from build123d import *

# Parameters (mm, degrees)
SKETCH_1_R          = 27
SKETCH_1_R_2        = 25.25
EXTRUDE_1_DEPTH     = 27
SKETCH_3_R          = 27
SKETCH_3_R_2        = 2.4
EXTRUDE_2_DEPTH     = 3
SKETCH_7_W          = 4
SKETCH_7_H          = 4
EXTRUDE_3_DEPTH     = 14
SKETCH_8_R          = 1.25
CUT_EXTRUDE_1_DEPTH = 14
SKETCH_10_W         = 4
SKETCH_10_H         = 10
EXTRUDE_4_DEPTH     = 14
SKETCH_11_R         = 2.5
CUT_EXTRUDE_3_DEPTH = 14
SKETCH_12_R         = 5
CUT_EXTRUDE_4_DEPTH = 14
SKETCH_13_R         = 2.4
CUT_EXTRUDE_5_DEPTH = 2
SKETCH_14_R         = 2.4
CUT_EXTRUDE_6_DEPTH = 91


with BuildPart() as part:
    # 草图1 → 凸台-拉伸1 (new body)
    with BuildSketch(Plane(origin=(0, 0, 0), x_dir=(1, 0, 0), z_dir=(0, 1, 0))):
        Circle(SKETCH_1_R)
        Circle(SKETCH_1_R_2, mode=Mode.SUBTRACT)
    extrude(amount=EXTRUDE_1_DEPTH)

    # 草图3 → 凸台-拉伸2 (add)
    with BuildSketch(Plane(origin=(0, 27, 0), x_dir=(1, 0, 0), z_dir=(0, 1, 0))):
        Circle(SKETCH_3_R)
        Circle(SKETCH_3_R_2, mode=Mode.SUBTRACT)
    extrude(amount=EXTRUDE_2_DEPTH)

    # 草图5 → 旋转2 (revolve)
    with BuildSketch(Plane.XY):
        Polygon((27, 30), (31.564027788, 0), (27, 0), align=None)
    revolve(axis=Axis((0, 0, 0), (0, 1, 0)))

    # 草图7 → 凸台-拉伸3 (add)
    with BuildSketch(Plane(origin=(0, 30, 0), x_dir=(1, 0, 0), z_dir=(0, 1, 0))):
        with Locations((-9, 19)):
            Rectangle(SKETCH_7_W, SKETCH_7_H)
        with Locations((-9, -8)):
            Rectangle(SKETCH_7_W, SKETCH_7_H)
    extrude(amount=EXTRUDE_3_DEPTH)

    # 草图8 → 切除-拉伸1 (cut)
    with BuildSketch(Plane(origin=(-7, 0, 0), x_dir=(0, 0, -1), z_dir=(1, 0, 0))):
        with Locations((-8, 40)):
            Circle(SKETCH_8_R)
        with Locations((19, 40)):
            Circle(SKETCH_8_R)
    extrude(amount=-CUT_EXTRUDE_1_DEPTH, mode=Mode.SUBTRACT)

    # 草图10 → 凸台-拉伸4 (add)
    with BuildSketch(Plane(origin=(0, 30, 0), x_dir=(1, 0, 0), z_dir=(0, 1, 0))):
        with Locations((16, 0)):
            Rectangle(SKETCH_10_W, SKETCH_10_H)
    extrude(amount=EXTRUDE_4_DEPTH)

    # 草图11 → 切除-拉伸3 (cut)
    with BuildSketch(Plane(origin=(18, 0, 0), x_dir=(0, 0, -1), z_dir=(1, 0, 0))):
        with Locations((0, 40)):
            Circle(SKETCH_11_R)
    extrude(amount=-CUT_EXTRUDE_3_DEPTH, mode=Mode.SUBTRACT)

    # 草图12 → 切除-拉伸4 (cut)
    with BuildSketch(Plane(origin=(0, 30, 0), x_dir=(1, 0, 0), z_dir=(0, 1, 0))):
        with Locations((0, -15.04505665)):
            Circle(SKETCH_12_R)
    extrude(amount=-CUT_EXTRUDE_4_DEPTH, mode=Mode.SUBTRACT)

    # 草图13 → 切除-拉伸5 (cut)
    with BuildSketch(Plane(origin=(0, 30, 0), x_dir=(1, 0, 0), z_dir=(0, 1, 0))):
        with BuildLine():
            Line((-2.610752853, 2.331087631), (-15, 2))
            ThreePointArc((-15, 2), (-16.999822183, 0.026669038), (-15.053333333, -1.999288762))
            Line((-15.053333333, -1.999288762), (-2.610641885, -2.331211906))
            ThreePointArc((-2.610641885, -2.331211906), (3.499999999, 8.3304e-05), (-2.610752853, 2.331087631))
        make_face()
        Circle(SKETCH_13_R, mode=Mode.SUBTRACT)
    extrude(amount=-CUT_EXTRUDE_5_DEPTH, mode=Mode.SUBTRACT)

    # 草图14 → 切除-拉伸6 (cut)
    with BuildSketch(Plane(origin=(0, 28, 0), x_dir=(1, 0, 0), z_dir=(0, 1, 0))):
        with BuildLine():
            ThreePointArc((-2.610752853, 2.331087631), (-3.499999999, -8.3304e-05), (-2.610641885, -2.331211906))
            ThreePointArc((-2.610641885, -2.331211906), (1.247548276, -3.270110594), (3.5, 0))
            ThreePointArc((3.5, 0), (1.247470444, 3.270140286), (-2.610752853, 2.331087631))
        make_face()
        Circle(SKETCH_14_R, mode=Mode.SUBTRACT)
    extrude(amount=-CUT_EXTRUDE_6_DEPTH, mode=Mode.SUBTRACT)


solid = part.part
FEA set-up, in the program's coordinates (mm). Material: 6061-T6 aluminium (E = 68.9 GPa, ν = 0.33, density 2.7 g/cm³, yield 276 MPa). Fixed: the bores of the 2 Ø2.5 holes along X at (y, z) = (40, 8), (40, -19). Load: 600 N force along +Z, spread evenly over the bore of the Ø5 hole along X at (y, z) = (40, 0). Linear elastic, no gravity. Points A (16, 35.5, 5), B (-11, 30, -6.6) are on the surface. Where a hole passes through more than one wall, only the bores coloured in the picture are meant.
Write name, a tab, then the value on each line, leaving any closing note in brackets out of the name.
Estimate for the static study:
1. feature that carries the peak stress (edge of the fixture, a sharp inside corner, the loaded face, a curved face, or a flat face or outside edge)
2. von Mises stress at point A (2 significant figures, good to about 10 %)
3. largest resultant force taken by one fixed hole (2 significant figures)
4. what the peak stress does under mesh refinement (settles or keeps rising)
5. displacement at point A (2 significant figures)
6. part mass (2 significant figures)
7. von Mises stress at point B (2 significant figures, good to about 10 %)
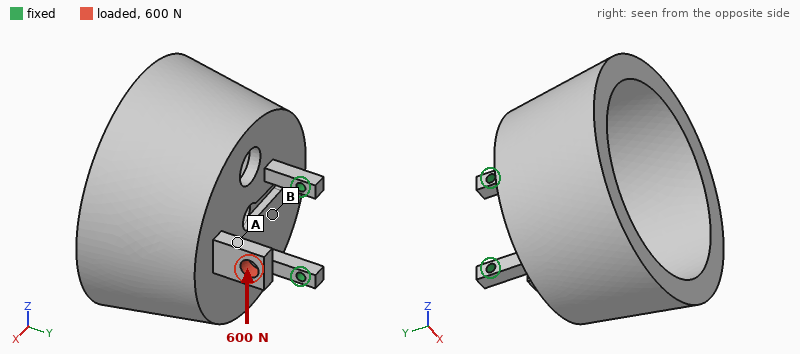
feature that carries the peak stress	edge of the fixture
von Mises stress at point A	58 MPa
largest resultant force taken by one fixed hole	620 N
what the peak stress does under mesh refinement	keeps rising
displacement at point A	0.18 mm
part mass	74 g
von Mises stress at point B	20 MPa
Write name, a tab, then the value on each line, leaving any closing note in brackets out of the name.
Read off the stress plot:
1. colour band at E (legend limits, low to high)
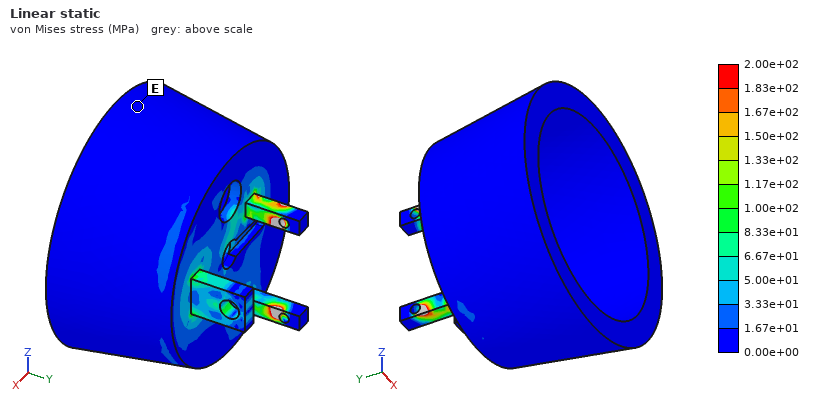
colour band at E	0.00e+00 to 1.67e+01 MPa
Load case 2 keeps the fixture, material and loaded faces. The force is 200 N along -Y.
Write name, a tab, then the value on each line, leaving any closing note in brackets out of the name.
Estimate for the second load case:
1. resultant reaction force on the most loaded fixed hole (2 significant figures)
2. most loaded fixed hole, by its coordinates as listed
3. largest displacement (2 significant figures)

resultant reaction force on the most loaded fixed hole	140 N
most loaded fixed hole, by its coordinates as listed	(40, 8)
largest displacement	1.0 mm
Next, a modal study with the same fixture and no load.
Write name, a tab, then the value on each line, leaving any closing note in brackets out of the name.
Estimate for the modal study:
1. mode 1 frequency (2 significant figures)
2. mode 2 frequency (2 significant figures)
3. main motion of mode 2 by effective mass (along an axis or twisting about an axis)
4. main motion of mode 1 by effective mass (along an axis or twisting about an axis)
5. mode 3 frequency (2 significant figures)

mode 1 frequency	330 Hz
mode 2 frequency	1100 Hz
main motion of mode 2 by effective mass	along Z
main motion of mode 1 by effective mass	along X
mode 3 frequency	1700 Hz
